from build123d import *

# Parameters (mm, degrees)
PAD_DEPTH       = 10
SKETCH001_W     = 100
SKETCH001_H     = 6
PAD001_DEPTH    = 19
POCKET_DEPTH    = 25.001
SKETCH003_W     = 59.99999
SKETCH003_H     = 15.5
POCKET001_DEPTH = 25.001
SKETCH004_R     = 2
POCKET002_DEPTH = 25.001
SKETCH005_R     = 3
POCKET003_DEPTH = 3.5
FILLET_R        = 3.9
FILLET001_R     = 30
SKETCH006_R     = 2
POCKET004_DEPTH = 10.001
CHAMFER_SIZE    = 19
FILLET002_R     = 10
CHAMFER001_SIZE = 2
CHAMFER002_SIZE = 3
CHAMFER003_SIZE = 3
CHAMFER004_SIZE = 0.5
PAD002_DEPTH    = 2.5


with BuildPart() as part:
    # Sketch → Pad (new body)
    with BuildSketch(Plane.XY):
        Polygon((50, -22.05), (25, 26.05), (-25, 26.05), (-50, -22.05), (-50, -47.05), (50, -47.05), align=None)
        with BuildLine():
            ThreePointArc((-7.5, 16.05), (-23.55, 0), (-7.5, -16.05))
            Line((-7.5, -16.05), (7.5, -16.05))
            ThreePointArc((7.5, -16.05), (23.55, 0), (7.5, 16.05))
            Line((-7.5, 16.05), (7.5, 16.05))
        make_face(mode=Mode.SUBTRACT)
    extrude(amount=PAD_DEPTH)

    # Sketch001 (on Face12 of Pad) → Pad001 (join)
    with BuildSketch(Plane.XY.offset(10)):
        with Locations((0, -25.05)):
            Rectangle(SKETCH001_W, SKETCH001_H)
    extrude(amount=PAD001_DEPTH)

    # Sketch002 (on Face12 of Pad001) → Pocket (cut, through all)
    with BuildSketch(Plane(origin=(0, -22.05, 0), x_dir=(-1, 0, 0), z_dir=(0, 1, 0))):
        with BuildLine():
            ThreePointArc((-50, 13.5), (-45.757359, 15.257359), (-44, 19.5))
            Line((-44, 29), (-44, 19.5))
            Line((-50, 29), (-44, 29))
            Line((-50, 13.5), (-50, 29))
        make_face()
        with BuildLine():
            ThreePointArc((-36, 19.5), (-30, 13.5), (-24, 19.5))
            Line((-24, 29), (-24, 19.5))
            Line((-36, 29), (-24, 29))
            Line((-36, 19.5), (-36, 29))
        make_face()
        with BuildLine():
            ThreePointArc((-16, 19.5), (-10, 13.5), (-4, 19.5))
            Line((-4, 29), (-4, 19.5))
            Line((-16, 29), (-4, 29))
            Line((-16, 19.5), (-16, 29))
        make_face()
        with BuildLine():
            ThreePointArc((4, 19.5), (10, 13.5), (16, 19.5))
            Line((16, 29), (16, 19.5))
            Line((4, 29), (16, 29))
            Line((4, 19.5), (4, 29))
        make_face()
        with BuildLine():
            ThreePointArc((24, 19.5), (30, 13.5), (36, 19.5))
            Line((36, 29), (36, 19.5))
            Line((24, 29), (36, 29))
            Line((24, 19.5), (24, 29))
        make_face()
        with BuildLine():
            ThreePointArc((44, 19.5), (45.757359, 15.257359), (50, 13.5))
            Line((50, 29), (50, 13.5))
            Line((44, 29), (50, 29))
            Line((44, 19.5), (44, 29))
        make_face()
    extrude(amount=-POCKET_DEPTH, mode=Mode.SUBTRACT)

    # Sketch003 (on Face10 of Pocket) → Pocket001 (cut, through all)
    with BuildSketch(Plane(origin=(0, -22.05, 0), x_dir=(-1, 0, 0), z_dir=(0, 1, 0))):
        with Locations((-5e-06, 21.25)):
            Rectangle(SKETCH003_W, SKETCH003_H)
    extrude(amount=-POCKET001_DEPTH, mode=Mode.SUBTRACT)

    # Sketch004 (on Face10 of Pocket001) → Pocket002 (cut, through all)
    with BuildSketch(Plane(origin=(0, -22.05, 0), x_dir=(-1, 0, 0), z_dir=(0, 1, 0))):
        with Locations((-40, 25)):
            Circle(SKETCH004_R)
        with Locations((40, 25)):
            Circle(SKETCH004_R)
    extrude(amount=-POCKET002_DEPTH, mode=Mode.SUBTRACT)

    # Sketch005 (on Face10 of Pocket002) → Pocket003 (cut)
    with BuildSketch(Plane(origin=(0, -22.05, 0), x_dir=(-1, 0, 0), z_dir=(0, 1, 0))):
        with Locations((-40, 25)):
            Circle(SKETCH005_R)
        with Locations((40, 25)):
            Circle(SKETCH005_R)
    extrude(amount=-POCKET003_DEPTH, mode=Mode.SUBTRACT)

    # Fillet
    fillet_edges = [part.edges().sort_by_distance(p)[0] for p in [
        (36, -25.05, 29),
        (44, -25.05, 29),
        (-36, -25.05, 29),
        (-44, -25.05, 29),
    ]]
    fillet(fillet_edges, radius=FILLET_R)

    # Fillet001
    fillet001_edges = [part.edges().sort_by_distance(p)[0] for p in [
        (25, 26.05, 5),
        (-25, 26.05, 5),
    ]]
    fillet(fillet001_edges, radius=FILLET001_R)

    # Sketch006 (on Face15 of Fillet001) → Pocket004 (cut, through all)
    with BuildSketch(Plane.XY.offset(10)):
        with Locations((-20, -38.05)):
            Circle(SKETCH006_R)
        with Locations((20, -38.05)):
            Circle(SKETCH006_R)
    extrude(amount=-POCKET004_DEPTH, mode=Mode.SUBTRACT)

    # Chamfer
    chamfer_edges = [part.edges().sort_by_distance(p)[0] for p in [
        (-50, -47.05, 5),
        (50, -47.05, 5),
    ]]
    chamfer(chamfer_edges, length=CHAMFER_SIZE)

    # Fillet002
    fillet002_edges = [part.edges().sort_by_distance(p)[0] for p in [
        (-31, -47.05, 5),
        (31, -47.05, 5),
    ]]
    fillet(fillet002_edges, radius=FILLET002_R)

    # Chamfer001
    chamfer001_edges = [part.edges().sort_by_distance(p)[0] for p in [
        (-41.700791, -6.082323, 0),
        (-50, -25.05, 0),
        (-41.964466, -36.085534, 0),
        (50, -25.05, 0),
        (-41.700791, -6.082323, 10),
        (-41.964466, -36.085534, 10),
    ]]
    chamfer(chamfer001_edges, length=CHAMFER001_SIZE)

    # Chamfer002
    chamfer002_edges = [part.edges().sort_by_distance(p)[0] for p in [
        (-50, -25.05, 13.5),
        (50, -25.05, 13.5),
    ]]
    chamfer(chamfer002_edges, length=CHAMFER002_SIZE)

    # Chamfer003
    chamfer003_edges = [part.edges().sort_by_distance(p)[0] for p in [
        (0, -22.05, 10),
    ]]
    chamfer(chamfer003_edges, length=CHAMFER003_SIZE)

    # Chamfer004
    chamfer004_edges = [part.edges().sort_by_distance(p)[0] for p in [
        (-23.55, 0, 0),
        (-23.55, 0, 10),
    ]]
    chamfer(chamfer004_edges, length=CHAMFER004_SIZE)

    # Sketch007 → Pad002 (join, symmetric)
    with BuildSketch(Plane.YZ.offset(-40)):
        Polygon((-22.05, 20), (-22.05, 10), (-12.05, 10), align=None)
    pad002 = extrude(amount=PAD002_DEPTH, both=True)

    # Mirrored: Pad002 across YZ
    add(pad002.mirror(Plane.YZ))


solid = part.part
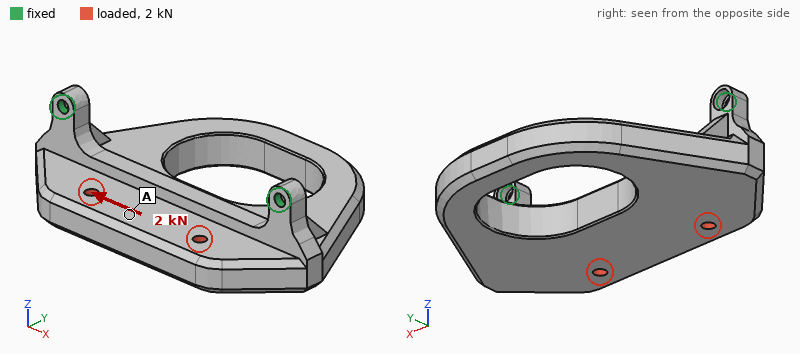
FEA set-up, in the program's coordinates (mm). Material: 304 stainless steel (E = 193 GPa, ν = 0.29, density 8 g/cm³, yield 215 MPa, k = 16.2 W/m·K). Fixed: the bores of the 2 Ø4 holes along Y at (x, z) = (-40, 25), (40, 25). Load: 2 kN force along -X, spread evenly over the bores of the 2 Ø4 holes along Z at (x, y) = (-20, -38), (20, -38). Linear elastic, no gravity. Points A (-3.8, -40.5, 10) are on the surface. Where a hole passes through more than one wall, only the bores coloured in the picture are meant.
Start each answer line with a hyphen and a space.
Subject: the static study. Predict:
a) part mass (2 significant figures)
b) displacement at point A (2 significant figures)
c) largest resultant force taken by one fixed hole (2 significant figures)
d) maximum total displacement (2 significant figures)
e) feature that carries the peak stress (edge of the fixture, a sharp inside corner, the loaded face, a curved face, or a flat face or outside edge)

- 370 g
- 15 µm
- 1.1 kN
- 17 µm
- edge of the fixture
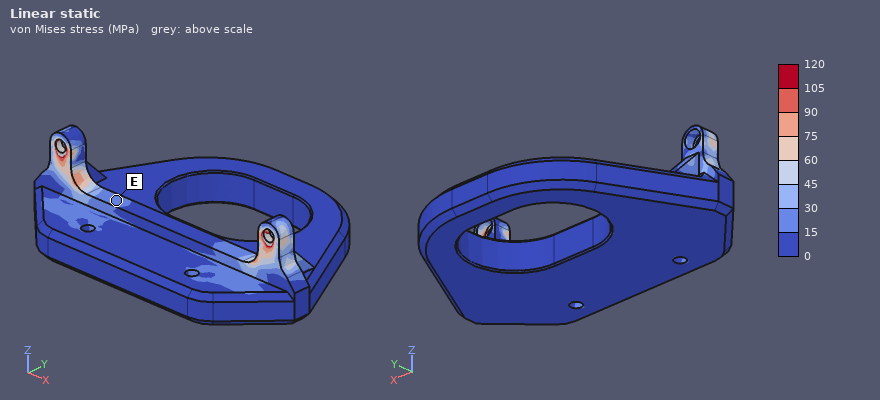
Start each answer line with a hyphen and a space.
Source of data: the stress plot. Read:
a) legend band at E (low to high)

- 15 to 30 MPa
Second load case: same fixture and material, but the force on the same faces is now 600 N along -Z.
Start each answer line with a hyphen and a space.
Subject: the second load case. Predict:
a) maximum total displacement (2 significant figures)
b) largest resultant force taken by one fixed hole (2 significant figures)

- 0.13 mm
- 350 N
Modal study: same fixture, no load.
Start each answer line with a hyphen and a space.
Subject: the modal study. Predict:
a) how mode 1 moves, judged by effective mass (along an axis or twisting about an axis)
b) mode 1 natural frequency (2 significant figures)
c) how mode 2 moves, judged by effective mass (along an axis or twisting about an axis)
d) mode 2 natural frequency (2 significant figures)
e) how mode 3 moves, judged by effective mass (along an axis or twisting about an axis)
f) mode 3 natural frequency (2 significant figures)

- along Y
- 550 Hz
- along X
- 2900 Hz
- along Y
- 3600 Hz
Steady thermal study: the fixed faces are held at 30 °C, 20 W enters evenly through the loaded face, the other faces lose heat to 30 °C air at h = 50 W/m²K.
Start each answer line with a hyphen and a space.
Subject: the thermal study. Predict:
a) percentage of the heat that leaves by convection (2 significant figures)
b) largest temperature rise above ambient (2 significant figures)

- 87 %
- 60 K
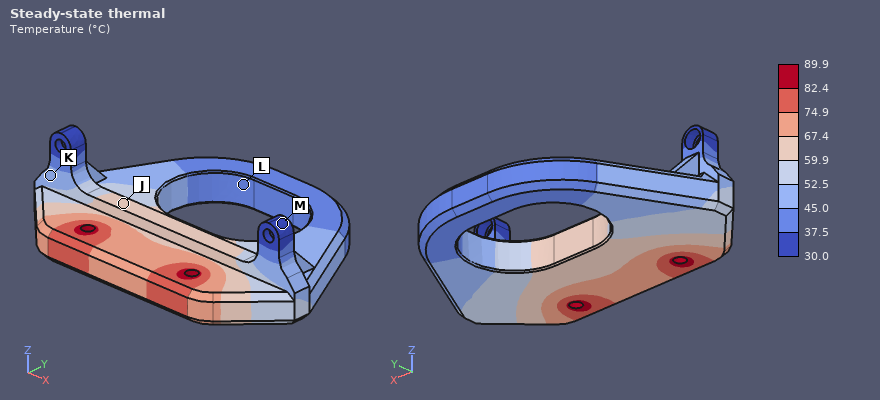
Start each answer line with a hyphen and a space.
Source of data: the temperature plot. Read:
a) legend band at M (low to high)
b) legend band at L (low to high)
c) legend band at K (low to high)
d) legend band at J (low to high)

- 30.0 to 37.5 °C
- 37.5 to 45.0 °C
- 45.0 to 52.5 °C
- 59.9 to 67.4 °C
